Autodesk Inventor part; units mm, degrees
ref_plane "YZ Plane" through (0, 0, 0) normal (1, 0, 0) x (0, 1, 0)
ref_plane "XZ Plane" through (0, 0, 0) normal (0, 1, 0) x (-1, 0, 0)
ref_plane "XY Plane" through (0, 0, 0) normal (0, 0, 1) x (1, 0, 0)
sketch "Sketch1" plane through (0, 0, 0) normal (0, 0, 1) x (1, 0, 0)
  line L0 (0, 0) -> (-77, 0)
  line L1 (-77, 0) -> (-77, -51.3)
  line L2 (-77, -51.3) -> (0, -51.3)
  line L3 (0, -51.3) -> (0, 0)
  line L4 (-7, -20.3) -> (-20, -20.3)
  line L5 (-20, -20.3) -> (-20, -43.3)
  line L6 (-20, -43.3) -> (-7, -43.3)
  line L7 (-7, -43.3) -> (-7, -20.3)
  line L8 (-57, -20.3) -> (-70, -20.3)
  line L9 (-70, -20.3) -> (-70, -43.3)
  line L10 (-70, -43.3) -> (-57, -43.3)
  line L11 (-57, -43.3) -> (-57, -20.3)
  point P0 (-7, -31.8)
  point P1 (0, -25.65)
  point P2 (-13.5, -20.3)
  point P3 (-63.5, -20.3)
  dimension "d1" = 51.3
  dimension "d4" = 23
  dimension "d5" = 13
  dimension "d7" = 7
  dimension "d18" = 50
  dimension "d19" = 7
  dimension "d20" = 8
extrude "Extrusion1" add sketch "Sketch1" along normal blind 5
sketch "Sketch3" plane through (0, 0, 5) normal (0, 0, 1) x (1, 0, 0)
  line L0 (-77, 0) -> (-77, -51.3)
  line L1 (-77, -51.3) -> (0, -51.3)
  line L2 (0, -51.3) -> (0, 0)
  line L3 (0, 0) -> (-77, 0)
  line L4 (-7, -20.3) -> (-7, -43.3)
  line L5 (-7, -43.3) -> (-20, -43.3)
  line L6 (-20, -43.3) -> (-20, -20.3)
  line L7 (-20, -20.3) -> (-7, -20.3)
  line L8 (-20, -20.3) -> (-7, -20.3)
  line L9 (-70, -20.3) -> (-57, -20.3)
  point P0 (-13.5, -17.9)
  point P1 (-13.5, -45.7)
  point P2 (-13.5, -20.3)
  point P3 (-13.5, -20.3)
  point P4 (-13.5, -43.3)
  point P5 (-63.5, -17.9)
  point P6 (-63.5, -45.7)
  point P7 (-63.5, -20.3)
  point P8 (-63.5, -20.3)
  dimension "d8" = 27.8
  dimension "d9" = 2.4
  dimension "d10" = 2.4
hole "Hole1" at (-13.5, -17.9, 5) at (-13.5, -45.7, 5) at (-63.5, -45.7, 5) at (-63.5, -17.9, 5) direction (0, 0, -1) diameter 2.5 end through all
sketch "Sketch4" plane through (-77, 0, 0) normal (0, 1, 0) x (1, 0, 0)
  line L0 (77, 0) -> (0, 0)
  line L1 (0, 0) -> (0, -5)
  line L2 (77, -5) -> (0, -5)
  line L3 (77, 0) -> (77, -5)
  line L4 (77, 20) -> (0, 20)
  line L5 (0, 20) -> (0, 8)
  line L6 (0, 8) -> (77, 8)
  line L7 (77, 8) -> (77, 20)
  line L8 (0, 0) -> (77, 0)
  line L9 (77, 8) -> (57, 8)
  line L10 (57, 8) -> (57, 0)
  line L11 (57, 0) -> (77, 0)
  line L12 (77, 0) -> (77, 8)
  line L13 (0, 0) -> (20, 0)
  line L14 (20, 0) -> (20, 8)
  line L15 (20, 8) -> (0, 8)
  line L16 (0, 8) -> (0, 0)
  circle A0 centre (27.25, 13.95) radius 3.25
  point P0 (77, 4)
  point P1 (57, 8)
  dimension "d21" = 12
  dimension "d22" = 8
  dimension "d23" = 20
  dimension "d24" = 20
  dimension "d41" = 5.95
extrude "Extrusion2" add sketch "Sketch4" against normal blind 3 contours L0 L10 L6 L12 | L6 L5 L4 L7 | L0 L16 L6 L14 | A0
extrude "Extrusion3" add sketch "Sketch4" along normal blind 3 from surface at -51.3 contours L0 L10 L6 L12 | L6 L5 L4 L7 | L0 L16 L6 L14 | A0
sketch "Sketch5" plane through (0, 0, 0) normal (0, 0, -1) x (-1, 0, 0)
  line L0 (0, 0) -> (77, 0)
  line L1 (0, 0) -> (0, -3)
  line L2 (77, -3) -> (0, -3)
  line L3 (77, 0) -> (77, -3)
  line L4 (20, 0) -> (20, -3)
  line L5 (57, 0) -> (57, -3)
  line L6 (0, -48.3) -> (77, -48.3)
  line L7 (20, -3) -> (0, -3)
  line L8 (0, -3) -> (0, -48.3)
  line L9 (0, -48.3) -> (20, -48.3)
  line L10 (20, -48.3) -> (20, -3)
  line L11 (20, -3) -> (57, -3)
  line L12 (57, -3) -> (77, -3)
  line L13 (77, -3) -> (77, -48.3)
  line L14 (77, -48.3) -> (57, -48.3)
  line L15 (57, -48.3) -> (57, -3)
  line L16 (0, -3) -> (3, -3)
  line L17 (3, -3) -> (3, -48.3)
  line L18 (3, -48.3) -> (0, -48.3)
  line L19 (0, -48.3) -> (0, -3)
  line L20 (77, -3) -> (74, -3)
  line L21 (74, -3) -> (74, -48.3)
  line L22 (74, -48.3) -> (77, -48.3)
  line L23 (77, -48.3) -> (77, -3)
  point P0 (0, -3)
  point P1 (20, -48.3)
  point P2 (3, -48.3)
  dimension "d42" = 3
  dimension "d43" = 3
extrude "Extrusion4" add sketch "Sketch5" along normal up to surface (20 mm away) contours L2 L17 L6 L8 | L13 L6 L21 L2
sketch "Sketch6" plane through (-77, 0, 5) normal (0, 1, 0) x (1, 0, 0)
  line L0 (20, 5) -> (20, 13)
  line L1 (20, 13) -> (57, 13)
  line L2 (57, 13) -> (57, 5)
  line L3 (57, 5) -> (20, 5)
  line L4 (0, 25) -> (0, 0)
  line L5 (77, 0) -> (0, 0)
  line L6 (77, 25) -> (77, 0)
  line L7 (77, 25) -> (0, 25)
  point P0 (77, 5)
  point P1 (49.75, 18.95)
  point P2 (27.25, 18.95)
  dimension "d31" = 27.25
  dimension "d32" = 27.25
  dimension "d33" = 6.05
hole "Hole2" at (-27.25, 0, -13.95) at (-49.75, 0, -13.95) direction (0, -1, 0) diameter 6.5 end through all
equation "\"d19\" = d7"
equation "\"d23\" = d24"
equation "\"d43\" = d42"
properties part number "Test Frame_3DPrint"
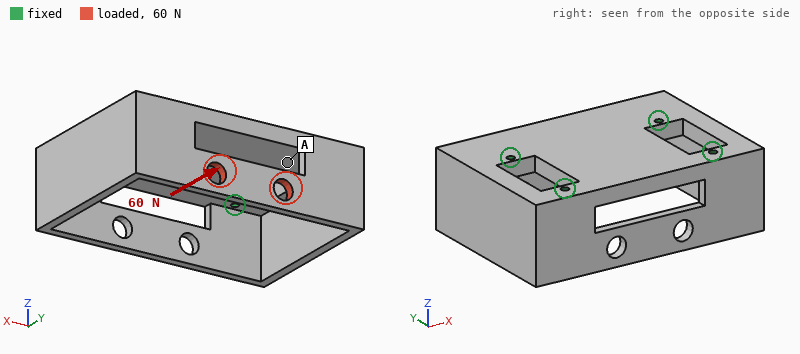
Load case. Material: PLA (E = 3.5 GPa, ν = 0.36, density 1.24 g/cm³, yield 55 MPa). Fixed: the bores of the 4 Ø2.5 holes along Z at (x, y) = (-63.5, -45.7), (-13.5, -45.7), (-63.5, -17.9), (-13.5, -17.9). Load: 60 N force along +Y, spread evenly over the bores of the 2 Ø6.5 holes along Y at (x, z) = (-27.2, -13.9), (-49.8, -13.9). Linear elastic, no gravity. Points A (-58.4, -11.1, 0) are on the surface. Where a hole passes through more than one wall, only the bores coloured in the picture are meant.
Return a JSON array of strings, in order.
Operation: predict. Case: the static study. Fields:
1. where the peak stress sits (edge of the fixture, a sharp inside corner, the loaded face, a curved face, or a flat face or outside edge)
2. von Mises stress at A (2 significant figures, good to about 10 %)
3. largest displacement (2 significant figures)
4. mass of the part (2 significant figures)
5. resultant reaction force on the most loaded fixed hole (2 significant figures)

["the loaded face", "1.8 MPa", "0.69 mm", "36 g", "32 N"]
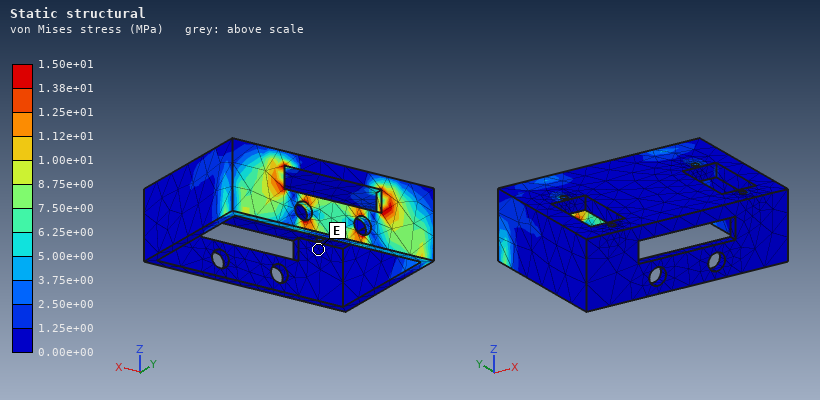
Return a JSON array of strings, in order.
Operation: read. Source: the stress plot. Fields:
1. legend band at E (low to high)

["0.00e+00 to 1.25e+00 MPa"]
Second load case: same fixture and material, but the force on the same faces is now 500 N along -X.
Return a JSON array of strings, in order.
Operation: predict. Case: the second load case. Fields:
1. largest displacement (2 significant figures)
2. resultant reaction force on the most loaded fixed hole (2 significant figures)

["0.55 mm", "300 N"]
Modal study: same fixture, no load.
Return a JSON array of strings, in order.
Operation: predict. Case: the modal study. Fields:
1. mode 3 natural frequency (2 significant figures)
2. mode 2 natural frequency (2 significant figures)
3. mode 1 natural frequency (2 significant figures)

["1700 Hz", "1300 Hz", "1300 Hz"]
